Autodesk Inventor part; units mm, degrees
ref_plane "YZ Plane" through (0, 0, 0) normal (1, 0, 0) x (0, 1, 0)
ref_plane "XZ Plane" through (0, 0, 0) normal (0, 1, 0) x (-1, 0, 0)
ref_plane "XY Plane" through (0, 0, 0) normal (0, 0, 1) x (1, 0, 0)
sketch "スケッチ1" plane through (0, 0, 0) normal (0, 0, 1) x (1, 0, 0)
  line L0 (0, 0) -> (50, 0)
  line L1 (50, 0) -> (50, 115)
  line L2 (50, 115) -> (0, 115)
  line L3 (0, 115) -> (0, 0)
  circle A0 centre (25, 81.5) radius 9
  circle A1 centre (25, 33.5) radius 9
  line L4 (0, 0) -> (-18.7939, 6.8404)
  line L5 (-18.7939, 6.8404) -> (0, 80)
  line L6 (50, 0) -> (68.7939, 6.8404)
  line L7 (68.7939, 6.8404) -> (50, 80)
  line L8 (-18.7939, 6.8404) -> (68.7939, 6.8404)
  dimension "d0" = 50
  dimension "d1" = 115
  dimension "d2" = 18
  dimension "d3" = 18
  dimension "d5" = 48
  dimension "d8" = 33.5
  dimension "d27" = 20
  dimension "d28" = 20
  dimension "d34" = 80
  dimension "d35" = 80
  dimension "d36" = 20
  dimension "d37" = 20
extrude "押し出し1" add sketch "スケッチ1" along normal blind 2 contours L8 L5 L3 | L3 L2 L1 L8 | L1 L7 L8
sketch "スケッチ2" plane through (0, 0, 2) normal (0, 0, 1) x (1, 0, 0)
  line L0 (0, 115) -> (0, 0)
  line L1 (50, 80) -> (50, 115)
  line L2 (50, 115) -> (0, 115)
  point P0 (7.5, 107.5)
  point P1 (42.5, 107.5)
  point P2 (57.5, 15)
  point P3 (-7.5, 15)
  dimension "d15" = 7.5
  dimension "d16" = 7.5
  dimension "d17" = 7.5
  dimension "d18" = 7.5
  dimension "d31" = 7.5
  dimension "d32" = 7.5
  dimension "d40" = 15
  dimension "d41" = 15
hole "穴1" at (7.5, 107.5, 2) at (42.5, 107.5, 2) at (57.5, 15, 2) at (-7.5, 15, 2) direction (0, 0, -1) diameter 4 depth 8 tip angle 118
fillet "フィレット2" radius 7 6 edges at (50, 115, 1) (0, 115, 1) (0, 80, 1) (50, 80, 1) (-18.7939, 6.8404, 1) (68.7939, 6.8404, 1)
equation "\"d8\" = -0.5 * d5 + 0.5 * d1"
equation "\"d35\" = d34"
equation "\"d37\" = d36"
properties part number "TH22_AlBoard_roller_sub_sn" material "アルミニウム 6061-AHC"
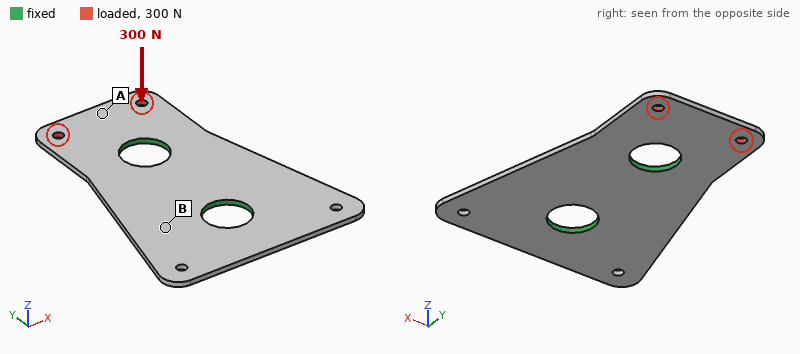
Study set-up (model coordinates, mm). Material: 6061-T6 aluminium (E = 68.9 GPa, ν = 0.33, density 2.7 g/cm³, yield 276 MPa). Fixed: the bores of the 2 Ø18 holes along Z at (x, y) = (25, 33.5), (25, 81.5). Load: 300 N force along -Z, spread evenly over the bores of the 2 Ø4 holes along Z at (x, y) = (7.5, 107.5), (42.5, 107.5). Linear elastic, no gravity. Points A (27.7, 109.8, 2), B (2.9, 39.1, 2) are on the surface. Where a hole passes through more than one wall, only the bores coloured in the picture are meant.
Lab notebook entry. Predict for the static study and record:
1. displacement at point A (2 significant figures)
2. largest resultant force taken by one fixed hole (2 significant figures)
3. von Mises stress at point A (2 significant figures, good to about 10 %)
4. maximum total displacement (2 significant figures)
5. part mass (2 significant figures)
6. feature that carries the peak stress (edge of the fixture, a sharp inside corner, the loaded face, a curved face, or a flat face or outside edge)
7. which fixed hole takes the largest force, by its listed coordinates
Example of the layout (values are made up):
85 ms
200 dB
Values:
0.34 mm
310 N
65 MPa
0.60 mm
33 g
a flat face or outside edge
(25, 81.5)
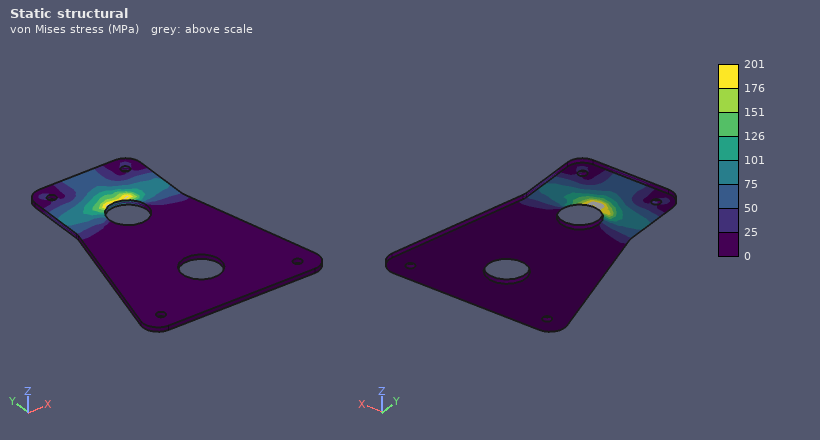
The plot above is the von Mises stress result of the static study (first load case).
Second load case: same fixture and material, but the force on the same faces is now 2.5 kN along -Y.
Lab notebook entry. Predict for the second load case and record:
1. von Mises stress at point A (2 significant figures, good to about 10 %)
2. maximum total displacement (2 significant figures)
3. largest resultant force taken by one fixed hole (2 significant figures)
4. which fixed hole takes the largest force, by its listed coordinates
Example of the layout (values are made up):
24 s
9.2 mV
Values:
16 MPa
18 µm
2.2 kN
(25, 81.5)
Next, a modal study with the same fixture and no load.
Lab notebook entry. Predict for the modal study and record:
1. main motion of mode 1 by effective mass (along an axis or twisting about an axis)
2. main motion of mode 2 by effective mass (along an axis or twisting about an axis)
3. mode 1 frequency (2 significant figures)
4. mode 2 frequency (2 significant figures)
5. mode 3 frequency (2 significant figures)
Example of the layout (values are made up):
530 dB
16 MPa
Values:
twisting about Y
along Z
1600 Hz
1700 Hz
2300 Hz
